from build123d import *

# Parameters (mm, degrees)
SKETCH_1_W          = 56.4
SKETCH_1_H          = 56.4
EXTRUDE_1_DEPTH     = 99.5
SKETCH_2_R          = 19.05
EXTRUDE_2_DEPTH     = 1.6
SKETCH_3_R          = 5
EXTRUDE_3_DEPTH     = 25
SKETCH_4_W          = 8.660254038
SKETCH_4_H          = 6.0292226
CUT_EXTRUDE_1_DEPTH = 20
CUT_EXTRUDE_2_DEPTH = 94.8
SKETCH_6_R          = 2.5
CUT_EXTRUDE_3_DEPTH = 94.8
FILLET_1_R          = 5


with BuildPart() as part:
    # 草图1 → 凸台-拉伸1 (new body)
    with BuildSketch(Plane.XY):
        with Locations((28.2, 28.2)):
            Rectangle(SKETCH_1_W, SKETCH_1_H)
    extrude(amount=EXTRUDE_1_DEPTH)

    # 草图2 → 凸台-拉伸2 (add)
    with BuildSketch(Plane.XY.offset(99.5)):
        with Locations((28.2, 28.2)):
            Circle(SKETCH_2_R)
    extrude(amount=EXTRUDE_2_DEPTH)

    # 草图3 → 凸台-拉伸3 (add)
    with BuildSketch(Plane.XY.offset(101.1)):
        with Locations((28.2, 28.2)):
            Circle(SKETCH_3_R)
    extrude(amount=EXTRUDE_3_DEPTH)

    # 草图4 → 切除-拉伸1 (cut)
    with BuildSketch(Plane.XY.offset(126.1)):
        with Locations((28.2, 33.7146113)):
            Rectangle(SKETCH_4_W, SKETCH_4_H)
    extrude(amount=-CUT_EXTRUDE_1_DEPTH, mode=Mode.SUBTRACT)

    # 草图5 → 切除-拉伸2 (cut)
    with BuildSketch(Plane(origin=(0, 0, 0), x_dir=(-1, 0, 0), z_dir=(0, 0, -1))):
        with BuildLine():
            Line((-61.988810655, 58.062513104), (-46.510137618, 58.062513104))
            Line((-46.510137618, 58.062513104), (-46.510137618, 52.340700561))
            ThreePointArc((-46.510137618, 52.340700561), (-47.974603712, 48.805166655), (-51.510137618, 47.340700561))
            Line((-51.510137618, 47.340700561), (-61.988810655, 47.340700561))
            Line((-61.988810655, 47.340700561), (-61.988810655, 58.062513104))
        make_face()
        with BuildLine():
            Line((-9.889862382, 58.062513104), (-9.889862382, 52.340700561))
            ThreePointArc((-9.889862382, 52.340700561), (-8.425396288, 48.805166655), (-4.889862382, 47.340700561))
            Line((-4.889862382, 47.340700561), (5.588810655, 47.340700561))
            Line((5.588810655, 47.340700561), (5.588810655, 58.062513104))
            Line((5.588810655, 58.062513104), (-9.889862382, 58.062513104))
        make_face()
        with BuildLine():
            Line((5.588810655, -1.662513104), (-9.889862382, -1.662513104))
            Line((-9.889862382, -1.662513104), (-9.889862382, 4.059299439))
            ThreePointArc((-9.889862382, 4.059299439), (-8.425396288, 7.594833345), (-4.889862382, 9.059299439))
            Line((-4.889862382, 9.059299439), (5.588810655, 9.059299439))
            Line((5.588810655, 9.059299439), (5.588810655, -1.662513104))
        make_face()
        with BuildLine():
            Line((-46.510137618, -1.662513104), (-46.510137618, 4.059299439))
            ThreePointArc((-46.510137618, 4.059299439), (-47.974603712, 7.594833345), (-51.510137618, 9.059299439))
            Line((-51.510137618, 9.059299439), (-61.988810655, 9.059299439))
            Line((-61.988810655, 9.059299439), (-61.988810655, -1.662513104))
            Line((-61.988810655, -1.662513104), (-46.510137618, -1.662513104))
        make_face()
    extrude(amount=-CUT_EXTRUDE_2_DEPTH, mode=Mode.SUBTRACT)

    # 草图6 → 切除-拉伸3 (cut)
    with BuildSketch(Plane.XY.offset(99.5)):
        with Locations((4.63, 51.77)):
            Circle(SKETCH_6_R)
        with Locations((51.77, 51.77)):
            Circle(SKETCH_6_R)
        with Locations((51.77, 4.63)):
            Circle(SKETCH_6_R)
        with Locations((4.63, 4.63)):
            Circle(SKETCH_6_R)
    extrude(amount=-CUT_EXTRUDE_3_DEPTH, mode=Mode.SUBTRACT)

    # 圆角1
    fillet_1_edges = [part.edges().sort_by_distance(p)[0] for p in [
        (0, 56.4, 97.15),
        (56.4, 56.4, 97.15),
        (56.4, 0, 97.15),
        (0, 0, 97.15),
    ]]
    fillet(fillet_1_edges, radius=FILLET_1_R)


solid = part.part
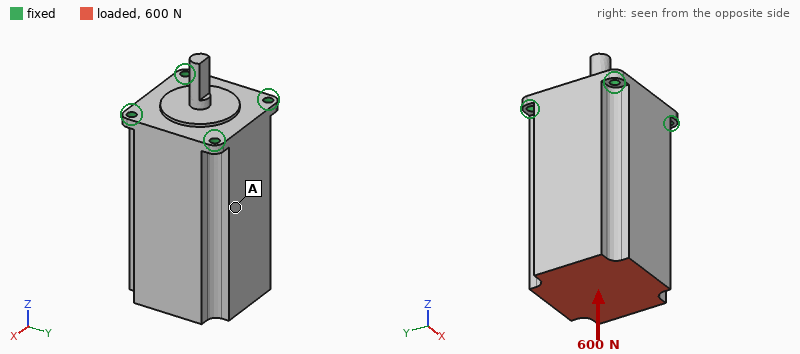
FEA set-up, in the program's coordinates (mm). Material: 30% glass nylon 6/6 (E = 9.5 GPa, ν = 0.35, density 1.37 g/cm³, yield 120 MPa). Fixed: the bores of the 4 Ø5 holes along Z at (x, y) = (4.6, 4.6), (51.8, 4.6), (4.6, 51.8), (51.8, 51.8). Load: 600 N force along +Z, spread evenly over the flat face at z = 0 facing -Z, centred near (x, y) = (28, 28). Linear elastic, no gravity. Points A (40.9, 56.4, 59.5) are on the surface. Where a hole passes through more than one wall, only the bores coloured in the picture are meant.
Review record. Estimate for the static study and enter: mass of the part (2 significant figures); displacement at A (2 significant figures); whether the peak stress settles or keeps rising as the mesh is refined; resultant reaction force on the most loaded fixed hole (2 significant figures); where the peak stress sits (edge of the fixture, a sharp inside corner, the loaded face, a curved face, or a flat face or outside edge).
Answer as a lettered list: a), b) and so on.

a) 390 g
b) 5.5 µm
c) keeps rising
d) 160 N
e) edge of the fixture
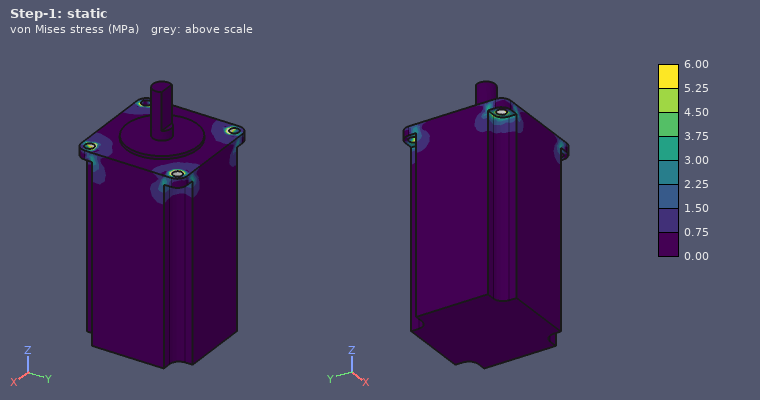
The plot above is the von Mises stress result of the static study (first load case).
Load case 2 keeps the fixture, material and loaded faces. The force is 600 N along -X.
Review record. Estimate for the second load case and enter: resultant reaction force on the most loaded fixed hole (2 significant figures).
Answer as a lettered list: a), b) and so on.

a) 700 N
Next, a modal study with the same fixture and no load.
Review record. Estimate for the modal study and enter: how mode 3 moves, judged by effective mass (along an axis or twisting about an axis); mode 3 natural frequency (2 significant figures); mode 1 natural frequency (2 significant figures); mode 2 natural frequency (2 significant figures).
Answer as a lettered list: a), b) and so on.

a) along Z
b) 2700 Hz
c) 980 Hz
d) 990 Hz
